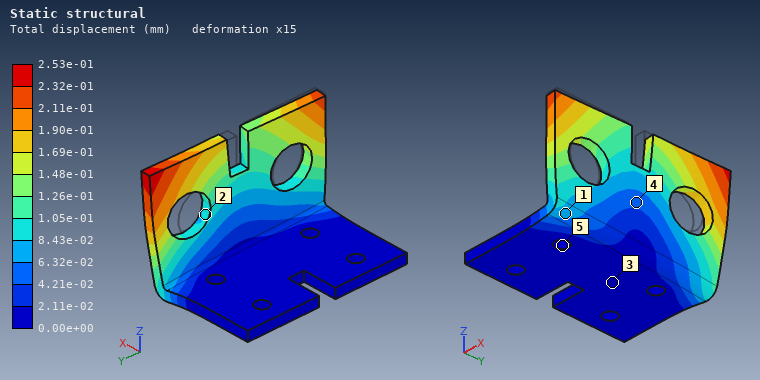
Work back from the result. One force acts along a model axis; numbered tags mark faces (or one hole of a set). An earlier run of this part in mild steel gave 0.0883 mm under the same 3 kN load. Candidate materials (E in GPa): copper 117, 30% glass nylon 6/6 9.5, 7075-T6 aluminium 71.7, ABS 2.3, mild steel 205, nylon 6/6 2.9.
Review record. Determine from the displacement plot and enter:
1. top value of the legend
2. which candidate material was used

2.53e-01 mm
7075-T6 aluminium
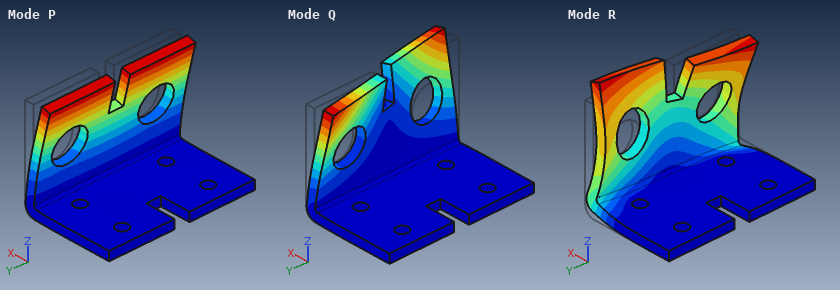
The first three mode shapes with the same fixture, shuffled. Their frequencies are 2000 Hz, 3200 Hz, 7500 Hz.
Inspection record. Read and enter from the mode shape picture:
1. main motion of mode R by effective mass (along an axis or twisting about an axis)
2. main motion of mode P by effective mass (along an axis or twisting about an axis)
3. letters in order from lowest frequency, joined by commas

along Y
along X
P, Q, R
